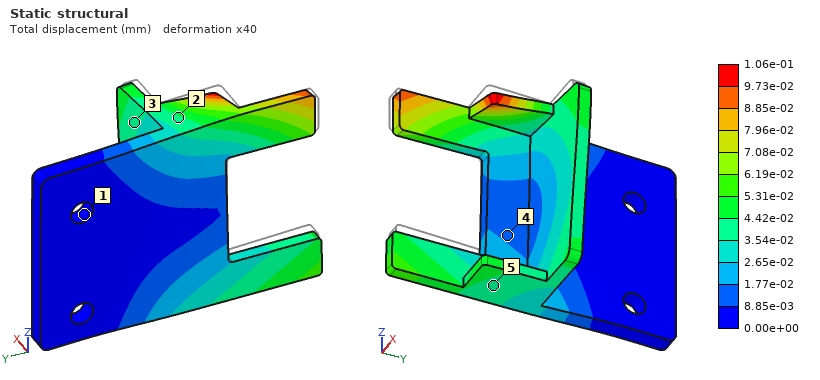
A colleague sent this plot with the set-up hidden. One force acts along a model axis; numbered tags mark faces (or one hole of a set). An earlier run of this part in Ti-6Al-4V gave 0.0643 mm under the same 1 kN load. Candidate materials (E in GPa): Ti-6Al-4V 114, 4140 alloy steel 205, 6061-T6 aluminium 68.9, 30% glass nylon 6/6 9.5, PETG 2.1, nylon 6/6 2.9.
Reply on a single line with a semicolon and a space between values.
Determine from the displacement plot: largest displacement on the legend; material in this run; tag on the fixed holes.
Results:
1.06e-01 mm; 6061-T6 aluminium; 1
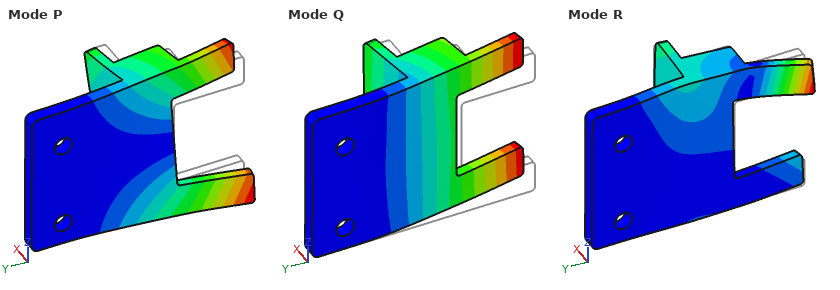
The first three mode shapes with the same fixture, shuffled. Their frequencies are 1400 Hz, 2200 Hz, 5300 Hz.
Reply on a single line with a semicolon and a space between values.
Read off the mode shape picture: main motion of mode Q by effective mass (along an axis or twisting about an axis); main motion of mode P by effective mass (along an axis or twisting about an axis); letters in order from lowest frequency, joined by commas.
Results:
along X; twisting about Y; Q, P, R
